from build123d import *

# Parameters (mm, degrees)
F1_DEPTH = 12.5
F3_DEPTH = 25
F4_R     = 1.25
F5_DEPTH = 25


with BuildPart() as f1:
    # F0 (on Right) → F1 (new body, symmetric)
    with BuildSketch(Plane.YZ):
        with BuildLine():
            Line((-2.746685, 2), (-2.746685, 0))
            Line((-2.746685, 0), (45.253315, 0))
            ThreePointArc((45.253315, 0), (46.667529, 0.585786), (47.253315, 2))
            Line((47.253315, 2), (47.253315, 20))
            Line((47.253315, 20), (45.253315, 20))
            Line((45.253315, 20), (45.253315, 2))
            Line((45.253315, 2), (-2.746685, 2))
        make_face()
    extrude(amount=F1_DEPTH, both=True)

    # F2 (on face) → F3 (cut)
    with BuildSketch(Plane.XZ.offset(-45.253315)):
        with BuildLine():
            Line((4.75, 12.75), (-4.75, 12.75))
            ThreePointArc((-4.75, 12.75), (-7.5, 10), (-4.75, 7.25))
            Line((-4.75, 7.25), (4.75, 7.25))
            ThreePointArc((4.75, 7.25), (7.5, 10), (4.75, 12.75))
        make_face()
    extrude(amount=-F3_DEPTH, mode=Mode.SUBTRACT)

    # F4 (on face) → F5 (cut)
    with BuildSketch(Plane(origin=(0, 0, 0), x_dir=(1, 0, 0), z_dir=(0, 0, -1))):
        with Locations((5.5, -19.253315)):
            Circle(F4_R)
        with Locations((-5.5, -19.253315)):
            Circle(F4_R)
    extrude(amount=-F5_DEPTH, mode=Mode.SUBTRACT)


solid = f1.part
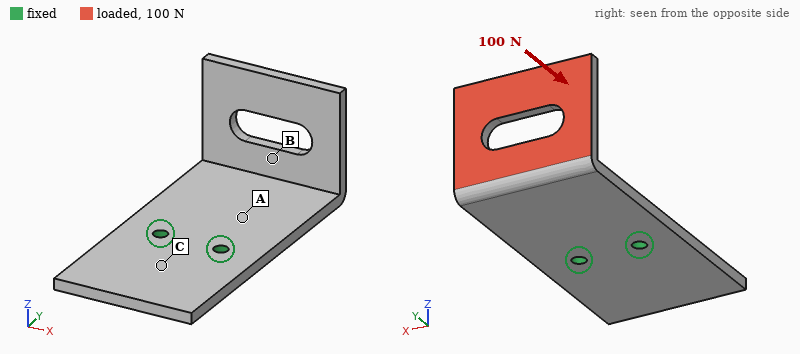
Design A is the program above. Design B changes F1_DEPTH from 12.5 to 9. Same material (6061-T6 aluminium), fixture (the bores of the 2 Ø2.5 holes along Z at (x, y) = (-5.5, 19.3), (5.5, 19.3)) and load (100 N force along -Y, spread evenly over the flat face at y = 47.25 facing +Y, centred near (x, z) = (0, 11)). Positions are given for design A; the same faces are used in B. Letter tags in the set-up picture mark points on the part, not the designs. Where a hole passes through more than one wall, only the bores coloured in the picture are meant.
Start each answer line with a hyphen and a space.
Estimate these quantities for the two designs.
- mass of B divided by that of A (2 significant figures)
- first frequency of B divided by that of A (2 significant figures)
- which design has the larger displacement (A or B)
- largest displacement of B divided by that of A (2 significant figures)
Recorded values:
- 0.71
- 1.0
- B
- 1.5
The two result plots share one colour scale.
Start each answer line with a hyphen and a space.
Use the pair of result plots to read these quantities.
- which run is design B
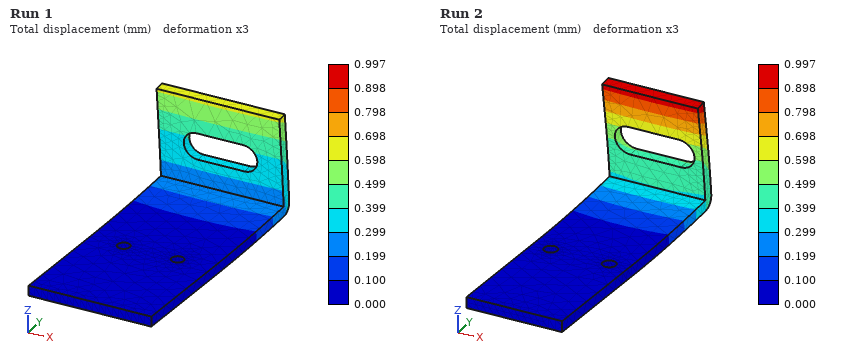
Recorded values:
- Run 2
